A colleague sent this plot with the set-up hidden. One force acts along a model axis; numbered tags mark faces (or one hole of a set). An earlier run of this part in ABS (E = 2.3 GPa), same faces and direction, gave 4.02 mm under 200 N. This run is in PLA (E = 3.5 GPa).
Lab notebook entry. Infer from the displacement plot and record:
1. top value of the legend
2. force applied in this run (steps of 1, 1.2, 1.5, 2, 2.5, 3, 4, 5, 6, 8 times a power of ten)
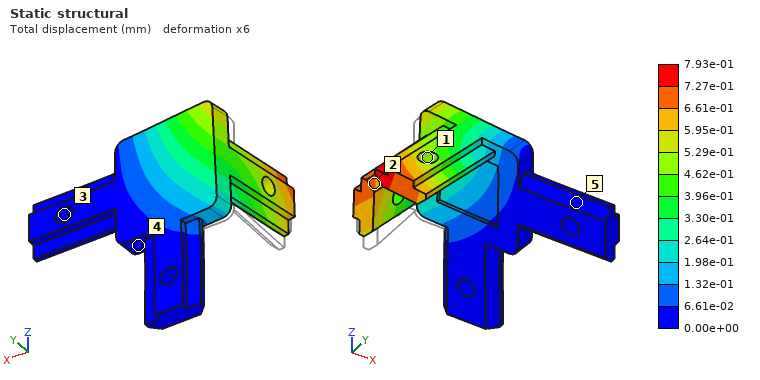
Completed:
7.93e-01 mm
60 N
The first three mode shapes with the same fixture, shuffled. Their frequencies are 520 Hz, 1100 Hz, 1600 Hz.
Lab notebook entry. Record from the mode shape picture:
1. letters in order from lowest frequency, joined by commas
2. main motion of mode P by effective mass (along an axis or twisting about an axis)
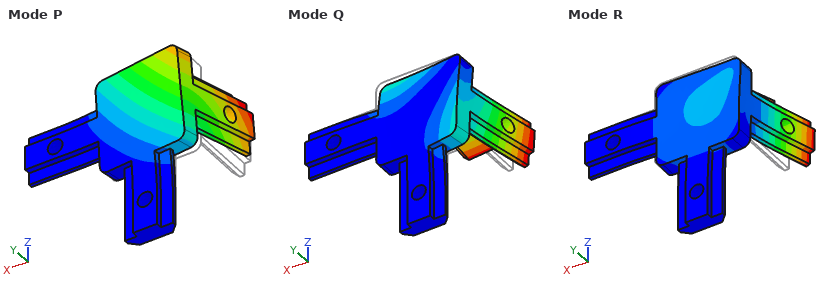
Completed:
P, Q, R
along Y
